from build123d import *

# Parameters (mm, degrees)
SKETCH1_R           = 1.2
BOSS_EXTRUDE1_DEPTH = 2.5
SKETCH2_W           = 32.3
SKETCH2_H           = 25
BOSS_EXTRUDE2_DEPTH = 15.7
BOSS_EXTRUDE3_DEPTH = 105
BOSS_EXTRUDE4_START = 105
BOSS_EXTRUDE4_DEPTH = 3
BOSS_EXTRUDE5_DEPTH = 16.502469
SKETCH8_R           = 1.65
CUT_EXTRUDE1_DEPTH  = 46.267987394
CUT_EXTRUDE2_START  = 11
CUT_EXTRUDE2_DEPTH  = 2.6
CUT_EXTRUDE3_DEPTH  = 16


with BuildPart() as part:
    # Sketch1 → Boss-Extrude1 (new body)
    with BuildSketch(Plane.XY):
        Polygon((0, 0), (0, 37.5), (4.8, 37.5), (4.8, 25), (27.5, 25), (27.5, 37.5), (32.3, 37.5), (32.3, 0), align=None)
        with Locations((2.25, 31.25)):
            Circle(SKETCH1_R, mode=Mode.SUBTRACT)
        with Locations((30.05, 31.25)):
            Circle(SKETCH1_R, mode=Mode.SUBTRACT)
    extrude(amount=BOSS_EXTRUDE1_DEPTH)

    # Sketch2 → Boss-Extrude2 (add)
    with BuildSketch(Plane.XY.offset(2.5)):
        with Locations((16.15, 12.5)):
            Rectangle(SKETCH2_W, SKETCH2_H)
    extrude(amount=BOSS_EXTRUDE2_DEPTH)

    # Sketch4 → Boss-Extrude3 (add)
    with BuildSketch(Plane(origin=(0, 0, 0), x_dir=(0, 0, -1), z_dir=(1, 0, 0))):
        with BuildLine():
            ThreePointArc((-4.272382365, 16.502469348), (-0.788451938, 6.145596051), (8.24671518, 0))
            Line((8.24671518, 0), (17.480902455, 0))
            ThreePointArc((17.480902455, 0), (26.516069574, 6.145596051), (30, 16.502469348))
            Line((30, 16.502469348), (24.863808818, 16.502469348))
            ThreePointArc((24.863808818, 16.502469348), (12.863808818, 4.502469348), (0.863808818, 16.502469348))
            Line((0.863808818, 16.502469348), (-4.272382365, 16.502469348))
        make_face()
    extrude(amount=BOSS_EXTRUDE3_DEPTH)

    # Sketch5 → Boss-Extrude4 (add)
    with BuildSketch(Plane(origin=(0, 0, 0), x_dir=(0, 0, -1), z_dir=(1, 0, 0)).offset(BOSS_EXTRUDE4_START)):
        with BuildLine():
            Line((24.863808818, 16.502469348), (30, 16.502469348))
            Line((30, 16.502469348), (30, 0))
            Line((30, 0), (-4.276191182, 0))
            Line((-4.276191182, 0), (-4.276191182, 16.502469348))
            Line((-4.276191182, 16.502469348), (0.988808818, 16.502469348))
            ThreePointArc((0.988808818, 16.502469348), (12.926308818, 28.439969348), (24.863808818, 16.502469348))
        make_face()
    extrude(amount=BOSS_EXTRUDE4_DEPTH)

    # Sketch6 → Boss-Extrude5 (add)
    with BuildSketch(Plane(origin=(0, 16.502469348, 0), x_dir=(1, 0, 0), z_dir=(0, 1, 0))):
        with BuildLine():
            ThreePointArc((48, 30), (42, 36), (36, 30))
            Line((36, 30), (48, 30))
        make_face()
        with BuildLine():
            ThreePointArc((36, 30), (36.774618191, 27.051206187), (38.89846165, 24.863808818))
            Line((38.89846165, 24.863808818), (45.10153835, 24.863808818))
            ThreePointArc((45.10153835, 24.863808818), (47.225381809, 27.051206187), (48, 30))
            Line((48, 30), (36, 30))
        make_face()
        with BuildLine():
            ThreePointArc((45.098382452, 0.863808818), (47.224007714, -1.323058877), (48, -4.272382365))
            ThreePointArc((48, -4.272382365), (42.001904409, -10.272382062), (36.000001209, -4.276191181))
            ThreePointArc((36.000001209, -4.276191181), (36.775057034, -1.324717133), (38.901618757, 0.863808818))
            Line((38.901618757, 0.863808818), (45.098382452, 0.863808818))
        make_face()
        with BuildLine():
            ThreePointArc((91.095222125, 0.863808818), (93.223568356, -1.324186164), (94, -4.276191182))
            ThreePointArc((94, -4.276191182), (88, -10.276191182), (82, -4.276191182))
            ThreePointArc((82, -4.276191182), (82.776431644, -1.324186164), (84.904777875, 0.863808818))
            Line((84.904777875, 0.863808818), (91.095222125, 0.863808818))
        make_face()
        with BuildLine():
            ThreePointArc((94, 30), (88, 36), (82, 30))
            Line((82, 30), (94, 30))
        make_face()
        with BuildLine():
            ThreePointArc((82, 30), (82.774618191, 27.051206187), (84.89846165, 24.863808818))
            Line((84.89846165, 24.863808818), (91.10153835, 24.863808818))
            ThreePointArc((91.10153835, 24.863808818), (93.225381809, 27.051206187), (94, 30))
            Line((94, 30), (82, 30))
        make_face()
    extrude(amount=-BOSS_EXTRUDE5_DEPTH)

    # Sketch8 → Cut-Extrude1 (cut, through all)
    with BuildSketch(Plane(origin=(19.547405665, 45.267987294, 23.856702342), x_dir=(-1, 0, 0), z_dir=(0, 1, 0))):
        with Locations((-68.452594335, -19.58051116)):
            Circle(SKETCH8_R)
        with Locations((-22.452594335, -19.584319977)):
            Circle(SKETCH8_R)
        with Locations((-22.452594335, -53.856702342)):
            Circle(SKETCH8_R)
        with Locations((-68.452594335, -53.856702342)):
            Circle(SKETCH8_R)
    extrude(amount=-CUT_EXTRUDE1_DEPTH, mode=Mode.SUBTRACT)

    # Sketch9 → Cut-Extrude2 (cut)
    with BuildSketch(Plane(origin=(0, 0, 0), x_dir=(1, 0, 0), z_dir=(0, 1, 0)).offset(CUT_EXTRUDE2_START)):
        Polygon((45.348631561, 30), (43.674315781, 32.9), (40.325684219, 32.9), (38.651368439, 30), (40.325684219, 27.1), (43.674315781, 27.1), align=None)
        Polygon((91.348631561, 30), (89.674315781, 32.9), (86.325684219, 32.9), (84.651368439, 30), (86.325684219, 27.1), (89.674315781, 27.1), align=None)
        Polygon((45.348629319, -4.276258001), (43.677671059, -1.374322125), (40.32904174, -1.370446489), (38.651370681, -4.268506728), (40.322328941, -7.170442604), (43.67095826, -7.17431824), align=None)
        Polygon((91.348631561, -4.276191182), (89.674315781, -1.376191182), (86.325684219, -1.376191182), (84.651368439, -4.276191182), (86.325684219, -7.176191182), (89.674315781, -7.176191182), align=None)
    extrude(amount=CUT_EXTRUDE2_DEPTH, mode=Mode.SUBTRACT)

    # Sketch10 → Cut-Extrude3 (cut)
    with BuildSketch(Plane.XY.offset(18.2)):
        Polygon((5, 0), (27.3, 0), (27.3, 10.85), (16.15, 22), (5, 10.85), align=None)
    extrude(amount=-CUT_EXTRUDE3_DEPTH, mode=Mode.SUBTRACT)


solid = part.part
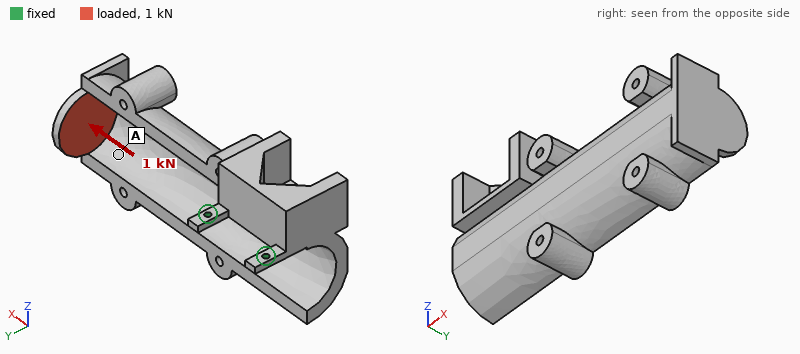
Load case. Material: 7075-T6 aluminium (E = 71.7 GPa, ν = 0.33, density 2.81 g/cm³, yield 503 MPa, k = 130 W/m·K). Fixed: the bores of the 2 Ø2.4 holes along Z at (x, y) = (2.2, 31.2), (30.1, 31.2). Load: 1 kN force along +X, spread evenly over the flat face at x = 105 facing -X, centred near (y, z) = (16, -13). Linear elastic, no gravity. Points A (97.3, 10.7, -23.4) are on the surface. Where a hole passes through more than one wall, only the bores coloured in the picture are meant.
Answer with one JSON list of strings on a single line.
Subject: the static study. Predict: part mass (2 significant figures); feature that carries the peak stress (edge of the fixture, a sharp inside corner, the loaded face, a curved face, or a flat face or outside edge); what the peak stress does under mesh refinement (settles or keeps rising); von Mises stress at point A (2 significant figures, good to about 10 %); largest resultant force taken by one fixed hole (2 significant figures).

["110 g", "edge of the fixture", "keeps rising", "21 MPa", "820 N"]
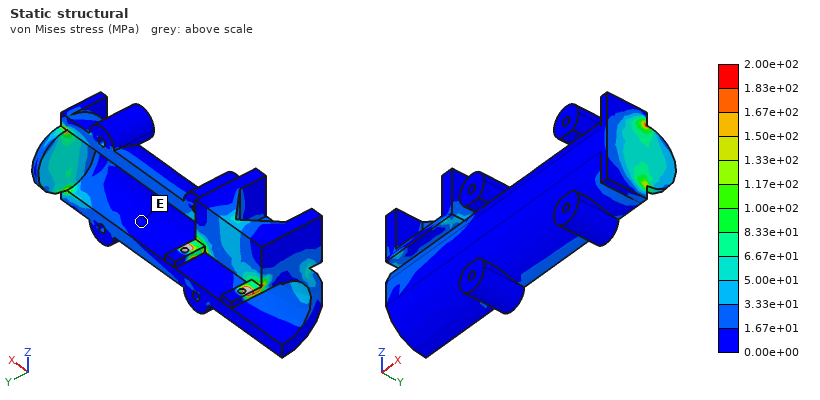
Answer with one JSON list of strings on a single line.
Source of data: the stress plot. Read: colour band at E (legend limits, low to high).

["0.00e+00 to 1.67e+01 MPa"]
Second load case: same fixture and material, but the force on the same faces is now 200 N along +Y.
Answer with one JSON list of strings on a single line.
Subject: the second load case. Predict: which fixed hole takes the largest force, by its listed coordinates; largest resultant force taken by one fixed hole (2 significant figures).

["(30.1, 31.2)", "740 N"]
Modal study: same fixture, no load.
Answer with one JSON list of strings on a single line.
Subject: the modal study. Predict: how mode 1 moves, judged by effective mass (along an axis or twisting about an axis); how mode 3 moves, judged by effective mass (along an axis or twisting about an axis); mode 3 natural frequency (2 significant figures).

["along Z", "along Y", "930 Hz"]
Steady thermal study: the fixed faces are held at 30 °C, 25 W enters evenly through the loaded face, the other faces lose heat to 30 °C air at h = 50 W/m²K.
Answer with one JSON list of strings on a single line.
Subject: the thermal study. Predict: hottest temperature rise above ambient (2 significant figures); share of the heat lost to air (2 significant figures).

["67 K", "84 %"]
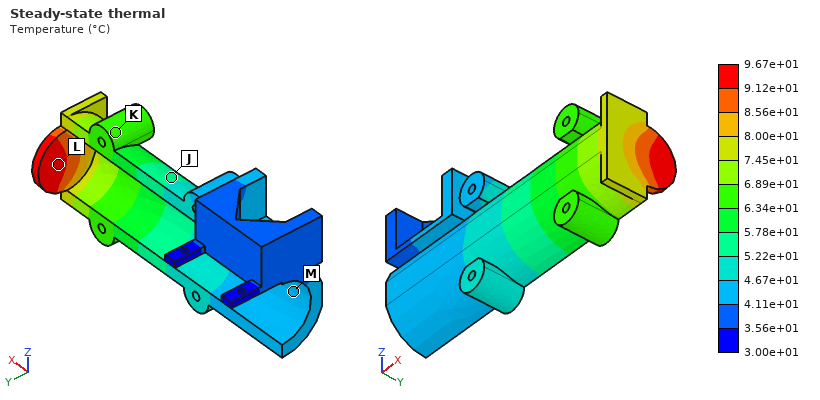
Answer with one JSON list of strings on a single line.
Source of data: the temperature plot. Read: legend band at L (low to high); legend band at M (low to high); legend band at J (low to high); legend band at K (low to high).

["9.12e+01 to 9.67e+01 °C", "4.11e+01 to 4.67e+01 °C", "5.22e+01 to 5.78e+01 °C", "6.34e+01 to 6.89e+01 °C"]
